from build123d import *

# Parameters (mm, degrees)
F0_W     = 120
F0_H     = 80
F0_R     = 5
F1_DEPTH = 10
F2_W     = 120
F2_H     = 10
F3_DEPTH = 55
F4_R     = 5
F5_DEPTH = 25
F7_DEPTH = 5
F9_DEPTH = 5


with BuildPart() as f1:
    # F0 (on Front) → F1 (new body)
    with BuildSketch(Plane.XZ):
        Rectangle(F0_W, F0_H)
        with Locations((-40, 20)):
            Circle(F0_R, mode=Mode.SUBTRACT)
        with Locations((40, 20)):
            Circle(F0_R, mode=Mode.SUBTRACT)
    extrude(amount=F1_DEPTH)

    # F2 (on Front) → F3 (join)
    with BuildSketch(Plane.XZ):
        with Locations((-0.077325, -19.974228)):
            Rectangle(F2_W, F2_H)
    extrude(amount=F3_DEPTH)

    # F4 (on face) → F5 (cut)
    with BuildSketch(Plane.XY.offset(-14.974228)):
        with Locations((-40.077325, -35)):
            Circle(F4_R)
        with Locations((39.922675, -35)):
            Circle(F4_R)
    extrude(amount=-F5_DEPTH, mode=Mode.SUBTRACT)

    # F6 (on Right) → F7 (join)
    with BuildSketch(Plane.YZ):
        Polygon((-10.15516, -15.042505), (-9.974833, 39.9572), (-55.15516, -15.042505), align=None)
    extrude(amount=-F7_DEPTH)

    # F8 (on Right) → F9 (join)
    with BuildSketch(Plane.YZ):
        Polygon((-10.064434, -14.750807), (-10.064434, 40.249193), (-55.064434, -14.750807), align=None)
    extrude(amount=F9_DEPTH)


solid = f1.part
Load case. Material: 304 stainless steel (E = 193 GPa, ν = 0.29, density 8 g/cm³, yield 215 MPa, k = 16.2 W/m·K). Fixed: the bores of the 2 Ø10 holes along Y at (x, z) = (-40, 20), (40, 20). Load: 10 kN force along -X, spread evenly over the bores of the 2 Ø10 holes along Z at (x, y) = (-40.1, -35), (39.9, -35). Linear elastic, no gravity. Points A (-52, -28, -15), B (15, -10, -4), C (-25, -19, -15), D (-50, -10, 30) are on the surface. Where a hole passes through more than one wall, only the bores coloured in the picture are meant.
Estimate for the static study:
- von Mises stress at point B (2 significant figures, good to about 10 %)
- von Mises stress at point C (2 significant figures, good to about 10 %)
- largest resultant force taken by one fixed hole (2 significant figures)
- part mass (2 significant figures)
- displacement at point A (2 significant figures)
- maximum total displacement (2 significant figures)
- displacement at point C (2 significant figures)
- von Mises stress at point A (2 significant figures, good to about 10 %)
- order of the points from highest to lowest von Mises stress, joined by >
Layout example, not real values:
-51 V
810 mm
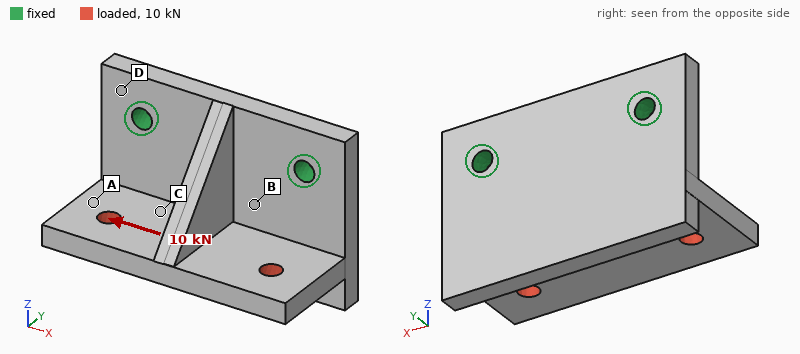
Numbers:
56 MPa
41 MPa
7.6 kN
1.3 kg
61 µm
91 µm
32 µm
30 MPa
B > C > A > D
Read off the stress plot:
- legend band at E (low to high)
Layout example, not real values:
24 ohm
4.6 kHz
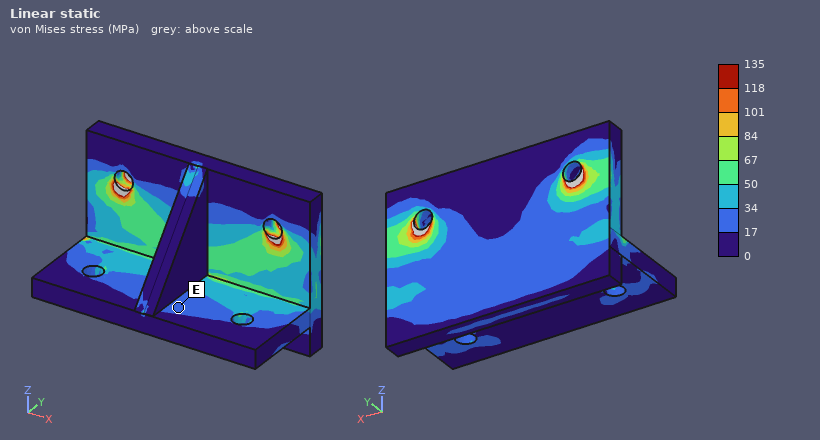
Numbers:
17 to 34 MPa
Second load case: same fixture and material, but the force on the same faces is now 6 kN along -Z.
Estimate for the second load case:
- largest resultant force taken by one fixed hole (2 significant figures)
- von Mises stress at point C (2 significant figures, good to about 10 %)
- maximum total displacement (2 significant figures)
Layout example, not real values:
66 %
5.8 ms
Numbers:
3.0 kN
36 MPa
0.17 mm
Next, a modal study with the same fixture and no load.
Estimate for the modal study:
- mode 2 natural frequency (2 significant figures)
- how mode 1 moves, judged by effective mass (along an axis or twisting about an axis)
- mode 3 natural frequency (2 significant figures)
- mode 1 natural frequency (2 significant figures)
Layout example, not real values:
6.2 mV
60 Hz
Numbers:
2200 Hz
along Y
3900 Hz
1300 Hz
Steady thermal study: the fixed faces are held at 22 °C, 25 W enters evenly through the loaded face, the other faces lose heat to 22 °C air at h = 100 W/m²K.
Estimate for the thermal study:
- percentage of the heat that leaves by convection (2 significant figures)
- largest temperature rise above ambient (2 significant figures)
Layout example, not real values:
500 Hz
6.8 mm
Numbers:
94 %
32 K
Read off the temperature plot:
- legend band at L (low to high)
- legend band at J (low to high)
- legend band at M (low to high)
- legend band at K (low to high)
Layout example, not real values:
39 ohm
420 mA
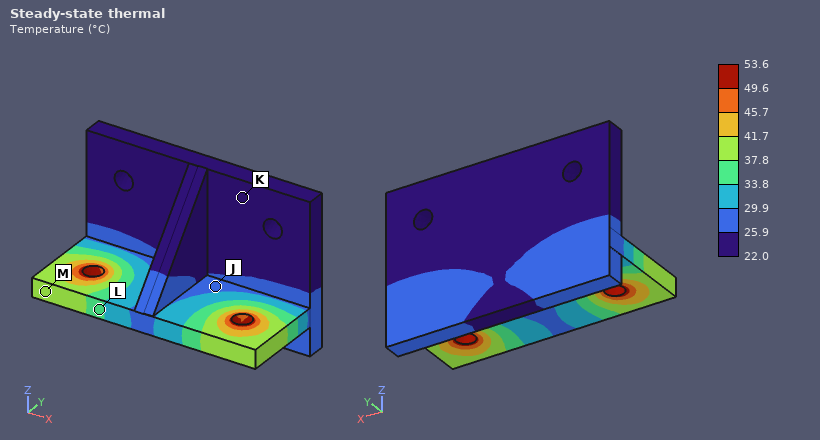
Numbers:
33.8 to 37.8 °C
25.9 to 29.9 °C
37.8 to 41.7 °C
22.0 to 25.9 °C
